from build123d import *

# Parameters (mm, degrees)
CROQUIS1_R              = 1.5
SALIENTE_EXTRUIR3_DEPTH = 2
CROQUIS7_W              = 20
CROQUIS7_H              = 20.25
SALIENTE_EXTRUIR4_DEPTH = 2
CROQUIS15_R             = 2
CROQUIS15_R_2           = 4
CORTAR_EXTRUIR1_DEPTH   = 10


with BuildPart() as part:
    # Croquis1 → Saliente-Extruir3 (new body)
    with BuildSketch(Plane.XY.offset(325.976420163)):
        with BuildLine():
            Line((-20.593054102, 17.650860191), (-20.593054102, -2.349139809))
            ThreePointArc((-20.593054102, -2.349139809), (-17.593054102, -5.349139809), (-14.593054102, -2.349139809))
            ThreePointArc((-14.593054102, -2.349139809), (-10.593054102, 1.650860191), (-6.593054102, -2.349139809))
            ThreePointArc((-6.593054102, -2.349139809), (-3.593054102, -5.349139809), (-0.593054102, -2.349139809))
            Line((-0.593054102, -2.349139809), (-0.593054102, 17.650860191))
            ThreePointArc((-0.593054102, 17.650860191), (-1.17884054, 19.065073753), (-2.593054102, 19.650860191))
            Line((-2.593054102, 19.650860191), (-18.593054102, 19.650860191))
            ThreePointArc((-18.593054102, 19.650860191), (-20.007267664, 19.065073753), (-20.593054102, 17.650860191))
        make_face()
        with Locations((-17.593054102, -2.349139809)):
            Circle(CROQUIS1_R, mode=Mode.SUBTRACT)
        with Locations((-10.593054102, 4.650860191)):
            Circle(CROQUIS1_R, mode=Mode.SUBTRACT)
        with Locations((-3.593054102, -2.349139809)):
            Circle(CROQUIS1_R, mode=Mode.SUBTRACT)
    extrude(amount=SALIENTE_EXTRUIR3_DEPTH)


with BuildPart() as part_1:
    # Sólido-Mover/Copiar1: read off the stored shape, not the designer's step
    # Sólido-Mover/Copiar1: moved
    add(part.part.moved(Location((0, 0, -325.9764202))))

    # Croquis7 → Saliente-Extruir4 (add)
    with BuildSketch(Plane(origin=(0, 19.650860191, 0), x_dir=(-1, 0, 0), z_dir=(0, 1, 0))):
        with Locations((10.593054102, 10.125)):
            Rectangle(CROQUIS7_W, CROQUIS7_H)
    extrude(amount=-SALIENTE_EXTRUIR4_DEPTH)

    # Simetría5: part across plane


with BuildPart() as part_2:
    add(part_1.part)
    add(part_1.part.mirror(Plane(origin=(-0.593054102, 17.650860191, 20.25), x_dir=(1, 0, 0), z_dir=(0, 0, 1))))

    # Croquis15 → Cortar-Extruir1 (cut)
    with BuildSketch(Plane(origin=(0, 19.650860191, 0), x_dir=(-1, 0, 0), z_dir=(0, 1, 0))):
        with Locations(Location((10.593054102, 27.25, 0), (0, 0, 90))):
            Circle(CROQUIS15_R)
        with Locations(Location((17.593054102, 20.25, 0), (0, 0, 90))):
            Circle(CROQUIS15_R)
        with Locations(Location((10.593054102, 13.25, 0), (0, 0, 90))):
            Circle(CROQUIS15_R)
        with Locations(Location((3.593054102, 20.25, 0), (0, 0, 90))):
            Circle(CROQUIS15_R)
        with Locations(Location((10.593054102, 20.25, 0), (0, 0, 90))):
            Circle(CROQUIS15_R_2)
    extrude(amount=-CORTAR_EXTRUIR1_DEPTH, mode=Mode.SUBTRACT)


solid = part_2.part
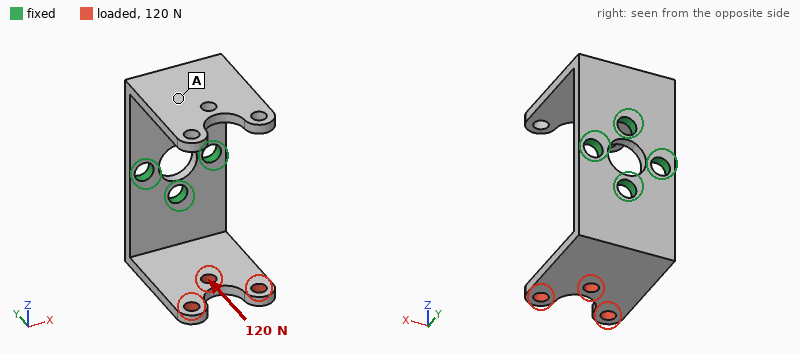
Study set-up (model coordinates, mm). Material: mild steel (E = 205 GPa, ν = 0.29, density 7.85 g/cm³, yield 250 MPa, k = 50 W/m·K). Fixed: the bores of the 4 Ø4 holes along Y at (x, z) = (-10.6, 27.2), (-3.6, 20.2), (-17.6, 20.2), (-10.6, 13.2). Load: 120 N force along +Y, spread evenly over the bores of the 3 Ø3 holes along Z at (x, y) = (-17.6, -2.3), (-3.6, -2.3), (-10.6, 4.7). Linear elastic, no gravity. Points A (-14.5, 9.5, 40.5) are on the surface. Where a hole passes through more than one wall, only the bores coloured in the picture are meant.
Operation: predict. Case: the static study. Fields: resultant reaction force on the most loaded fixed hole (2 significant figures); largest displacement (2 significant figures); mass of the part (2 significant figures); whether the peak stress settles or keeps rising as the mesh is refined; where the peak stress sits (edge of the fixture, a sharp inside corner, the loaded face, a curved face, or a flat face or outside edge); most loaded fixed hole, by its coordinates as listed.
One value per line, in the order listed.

180 N
74 µm
23 g
keeps rising
edge of the fixture
(-10.6, 13.2)
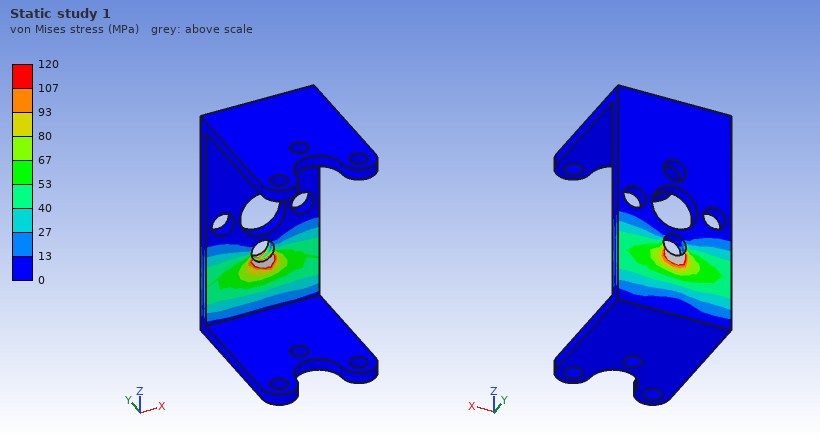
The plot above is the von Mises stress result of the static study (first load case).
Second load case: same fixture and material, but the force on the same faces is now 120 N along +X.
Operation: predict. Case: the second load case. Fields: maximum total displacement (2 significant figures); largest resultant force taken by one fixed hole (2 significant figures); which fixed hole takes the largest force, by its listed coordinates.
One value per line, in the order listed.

0.12 mm
130 N
(-10.6, 13.2)
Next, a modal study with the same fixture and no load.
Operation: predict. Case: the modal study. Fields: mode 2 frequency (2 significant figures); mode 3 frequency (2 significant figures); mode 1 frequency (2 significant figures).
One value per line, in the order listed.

2100 Hz
3100 Hz
2100 Hz
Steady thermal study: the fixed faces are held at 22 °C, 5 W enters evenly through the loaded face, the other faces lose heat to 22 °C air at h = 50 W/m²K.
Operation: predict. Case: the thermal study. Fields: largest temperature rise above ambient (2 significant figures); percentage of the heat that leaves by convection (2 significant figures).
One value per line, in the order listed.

62 K
42 %
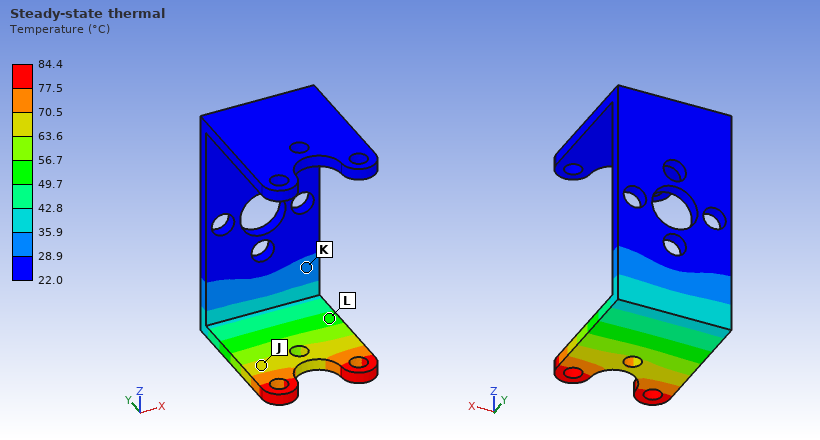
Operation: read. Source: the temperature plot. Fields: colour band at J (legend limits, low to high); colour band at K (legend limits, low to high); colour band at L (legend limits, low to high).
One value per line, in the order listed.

63.6 to 70.5 °C
28.9 to 35.9 °C
49.7 to 56.7 °C
